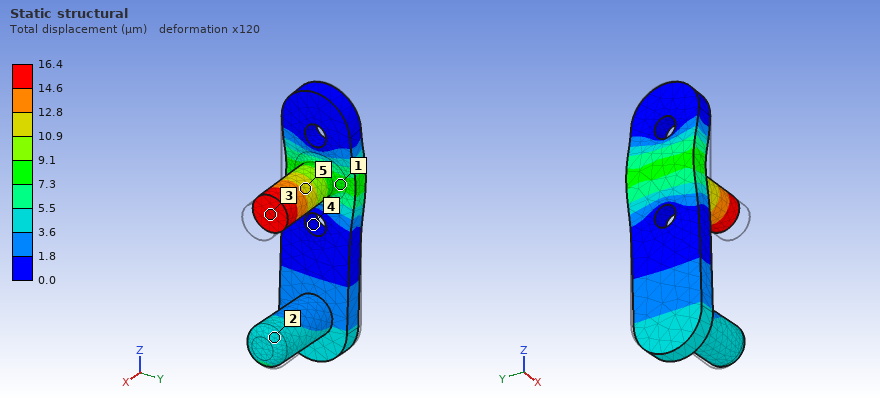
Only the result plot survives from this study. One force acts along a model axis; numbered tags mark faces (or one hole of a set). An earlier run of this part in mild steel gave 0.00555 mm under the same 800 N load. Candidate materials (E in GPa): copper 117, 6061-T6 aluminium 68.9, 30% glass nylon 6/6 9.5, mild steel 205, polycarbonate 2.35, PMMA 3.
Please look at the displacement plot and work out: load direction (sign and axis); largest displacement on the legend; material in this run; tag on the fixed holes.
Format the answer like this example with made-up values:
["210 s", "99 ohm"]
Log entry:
["-X", "16.4 µm", "6061-T6 aluminium", "4"]
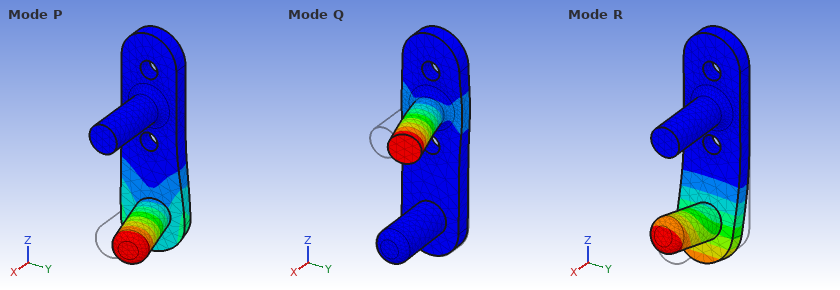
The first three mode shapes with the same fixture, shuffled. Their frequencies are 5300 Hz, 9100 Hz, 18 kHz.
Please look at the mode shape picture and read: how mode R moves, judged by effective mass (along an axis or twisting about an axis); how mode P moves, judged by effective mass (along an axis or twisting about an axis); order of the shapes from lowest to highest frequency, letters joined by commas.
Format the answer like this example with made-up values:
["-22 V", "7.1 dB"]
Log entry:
["along X", "along Y", "R, P, Q"]
